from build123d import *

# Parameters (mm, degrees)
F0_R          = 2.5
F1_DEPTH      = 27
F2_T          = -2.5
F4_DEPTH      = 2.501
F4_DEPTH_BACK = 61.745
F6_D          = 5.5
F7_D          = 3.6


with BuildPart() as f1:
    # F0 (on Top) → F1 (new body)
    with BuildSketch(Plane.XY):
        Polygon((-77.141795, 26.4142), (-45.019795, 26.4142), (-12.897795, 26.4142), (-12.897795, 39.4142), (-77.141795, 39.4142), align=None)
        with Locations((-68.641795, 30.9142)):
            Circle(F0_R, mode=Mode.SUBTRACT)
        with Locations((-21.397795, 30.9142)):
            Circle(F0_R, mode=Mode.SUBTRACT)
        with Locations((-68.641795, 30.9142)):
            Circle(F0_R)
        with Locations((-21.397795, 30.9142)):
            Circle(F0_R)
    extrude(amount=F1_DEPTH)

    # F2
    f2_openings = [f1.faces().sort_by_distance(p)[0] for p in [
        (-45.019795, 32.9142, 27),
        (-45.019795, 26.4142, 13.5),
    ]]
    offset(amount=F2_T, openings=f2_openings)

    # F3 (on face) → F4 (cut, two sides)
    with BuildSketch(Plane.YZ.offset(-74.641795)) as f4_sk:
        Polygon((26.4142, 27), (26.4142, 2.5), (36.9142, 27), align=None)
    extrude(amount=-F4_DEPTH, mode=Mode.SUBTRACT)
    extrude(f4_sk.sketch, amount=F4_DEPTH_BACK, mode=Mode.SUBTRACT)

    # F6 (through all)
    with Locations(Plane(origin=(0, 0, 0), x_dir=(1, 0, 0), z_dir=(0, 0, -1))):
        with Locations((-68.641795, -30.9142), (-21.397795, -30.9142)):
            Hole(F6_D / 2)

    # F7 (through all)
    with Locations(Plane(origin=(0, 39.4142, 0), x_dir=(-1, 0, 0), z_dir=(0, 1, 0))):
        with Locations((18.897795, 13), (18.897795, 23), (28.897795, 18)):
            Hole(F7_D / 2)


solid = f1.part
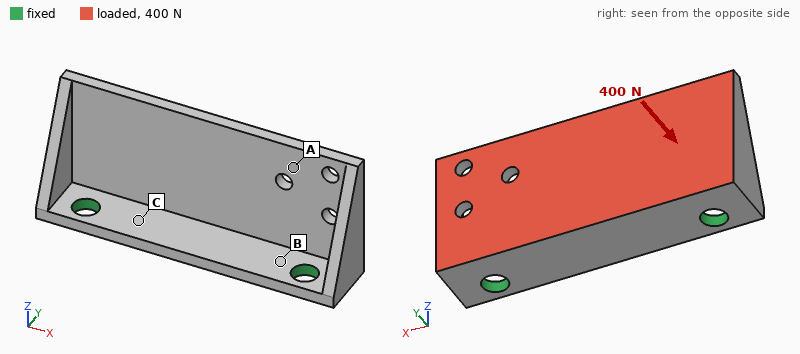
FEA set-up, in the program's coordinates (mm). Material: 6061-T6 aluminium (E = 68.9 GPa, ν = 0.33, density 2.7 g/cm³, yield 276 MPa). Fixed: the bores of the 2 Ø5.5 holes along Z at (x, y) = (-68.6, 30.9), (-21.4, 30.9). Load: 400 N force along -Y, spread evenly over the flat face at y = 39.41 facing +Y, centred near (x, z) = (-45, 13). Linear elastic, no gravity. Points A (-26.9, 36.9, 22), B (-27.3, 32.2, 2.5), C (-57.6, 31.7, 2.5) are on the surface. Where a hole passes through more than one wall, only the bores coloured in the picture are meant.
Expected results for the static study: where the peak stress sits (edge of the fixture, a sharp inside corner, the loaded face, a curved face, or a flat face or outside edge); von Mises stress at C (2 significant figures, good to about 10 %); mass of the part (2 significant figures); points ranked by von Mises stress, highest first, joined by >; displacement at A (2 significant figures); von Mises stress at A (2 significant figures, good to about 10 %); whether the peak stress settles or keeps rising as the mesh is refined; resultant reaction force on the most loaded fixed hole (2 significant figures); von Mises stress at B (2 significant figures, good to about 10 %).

edge of the fixture
33 MPa
17 g
B > C > A
0.11 mm
19 MPa
keeps rising
210 N
45 MPa
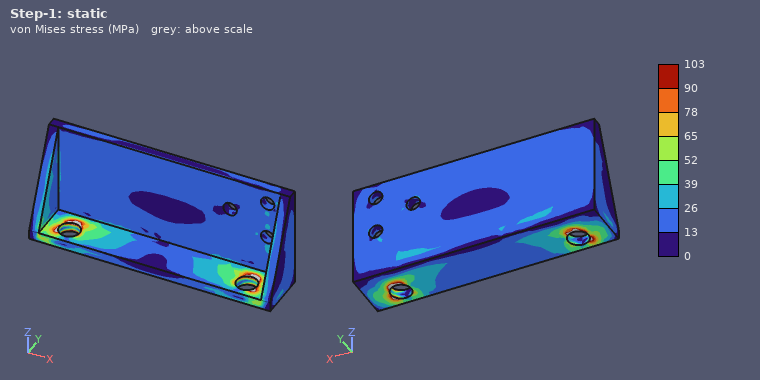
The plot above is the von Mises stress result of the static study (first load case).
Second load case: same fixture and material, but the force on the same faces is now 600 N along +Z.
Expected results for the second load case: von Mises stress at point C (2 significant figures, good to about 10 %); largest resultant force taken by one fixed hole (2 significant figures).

14 MPa
310 N
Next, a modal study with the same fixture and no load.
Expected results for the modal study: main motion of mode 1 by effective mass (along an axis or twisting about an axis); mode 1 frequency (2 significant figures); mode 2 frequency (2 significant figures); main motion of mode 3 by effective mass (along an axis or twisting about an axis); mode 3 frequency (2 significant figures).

along Y
2800 Hz
4900 Hz
along Z
7600 Hz
